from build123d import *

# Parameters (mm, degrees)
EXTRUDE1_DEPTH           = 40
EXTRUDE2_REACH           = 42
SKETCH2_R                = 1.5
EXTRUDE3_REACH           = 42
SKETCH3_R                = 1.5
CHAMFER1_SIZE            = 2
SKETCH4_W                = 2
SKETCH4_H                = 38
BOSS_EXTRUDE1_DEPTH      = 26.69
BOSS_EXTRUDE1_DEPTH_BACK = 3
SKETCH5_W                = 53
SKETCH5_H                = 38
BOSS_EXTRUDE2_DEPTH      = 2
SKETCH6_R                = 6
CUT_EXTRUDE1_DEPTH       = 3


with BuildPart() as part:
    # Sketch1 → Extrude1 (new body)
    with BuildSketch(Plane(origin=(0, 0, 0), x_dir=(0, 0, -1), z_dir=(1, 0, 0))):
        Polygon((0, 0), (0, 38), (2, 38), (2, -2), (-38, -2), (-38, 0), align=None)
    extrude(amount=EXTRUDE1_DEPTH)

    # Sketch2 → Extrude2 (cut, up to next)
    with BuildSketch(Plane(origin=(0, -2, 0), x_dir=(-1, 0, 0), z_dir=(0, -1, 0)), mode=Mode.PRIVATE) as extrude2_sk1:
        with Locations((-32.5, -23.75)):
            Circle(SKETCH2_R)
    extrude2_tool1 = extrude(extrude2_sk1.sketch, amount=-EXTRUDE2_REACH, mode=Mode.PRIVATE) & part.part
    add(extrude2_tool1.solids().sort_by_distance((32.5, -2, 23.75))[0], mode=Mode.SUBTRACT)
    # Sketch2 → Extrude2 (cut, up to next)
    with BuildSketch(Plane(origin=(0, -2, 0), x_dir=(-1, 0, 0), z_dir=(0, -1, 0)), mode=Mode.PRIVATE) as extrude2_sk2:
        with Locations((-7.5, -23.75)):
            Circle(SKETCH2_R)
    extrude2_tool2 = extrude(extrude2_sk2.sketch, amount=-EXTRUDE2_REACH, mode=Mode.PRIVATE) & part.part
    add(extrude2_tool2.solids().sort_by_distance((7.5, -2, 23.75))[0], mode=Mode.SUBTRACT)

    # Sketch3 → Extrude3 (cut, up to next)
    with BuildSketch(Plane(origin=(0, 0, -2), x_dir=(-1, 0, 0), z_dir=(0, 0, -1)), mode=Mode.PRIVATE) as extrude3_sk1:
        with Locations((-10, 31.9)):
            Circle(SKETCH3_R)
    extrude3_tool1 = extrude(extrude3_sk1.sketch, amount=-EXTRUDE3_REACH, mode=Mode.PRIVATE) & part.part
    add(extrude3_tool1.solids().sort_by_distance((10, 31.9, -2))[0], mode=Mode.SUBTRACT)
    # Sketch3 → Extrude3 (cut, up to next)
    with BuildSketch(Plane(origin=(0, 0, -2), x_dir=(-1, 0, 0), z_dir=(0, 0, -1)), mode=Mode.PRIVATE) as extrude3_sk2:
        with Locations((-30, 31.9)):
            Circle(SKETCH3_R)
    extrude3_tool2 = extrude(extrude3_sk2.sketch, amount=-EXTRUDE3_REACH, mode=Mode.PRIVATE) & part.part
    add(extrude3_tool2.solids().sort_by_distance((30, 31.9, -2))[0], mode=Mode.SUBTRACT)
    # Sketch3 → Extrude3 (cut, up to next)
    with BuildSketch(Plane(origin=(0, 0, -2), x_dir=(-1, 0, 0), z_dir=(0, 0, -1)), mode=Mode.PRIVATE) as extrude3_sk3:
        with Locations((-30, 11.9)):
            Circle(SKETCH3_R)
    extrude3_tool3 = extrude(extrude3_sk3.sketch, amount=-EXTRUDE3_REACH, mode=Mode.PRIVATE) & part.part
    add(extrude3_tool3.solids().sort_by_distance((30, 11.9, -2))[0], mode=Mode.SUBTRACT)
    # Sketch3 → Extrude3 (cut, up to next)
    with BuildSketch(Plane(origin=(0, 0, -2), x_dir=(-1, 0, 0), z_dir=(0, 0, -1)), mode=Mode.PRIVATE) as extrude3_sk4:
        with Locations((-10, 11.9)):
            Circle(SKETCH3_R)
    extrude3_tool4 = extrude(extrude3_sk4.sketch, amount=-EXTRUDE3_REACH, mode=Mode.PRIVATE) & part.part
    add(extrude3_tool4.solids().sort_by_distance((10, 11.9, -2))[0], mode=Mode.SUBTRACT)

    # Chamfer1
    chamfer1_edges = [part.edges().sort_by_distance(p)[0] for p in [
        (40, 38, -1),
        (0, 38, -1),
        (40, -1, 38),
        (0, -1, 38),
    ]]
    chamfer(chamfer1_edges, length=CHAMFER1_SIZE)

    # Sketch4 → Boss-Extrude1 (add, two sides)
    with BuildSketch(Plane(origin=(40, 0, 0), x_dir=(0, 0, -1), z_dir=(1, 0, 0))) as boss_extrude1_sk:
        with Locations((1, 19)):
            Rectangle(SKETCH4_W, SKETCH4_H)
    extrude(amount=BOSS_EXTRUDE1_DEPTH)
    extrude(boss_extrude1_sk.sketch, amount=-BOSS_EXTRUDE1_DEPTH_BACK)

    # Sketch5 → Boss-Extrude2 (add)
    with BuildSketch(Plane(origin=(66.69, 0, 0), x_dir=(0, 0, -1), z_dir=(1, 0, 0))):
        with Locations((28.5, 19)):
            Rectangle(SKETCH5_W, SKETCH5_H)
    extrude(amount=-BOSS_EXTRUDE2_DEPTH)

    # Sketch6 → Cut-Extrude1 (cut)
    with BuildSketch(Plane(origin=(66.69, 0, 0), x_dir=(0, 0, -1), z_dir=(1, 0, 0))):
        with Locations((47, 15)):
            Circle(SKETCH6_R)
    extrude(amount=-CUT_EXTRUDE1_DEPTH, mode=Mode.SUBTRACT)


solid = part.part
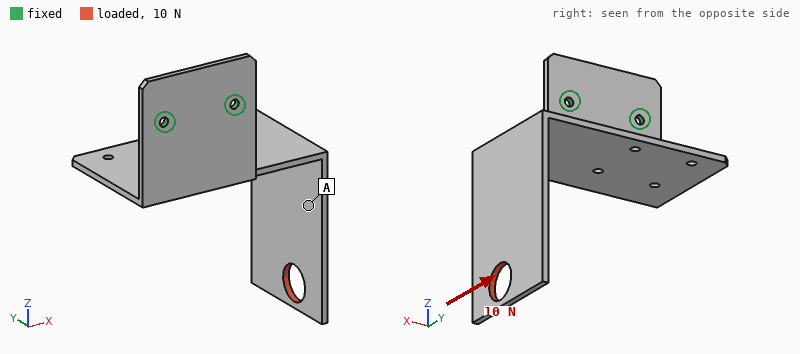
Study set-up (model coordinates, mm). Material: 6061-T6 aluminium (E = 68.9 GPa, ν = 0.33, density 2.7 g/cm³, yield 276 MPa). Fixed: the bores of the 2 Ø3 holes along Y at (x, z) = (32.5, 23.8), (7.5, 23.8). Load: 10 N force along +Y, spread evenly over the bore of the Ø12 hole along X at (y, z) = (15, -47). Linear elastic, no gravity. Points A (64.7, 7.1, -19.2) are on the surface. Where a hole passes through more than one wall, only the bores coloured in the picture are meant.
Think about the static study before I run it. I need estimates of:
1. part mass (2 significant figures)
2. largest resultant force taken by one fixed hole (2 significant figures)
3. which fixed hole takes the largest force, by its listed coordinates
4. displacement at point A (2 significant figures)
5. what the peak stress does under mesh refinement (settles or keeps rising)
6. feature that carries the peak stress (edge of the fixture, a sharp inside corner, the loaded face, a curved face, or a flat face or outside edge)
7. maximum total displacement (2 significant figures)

32 g
21 N
(32.5, 23.8)
0.51 mm
keeps rising
edge of the fixture
1.2 mm
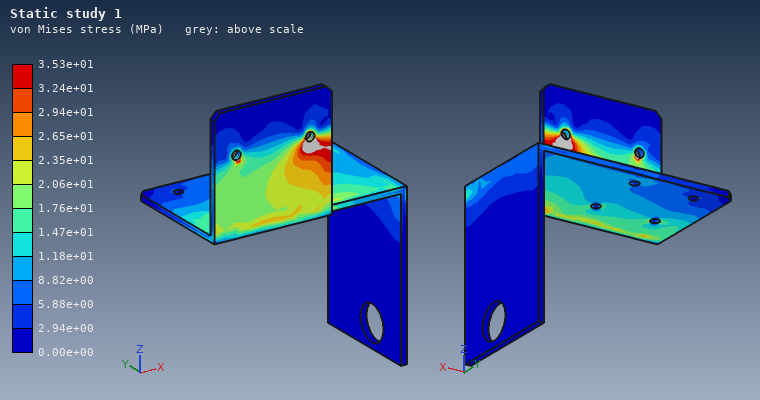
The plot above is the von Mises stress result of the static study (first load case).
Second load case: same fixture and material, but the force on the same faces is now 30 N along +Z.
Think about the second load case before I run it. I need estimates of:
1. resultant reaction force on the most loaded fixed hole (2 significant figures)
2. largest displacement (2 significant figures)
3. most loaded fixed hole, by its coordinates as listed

68 N
1.3 mm
(32.5, 23.8)
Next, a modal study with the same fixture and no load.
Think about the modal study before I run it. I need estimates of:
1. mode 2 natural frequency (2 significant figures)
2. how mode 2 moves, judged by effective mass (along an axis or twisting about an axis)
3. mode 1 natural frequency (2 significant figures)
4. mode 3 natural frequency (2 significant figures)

280 Hz
along X
180 Hz
560 Hz
